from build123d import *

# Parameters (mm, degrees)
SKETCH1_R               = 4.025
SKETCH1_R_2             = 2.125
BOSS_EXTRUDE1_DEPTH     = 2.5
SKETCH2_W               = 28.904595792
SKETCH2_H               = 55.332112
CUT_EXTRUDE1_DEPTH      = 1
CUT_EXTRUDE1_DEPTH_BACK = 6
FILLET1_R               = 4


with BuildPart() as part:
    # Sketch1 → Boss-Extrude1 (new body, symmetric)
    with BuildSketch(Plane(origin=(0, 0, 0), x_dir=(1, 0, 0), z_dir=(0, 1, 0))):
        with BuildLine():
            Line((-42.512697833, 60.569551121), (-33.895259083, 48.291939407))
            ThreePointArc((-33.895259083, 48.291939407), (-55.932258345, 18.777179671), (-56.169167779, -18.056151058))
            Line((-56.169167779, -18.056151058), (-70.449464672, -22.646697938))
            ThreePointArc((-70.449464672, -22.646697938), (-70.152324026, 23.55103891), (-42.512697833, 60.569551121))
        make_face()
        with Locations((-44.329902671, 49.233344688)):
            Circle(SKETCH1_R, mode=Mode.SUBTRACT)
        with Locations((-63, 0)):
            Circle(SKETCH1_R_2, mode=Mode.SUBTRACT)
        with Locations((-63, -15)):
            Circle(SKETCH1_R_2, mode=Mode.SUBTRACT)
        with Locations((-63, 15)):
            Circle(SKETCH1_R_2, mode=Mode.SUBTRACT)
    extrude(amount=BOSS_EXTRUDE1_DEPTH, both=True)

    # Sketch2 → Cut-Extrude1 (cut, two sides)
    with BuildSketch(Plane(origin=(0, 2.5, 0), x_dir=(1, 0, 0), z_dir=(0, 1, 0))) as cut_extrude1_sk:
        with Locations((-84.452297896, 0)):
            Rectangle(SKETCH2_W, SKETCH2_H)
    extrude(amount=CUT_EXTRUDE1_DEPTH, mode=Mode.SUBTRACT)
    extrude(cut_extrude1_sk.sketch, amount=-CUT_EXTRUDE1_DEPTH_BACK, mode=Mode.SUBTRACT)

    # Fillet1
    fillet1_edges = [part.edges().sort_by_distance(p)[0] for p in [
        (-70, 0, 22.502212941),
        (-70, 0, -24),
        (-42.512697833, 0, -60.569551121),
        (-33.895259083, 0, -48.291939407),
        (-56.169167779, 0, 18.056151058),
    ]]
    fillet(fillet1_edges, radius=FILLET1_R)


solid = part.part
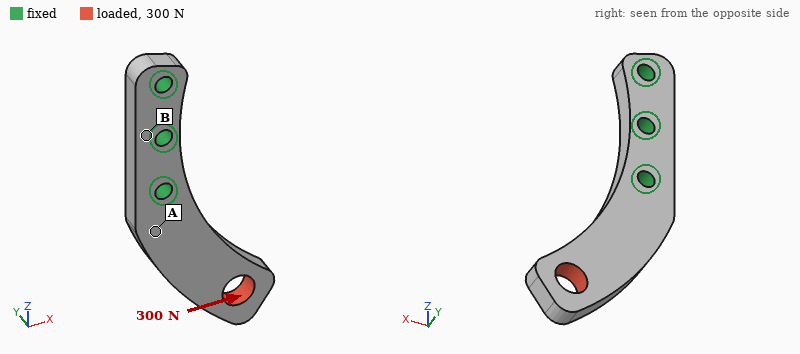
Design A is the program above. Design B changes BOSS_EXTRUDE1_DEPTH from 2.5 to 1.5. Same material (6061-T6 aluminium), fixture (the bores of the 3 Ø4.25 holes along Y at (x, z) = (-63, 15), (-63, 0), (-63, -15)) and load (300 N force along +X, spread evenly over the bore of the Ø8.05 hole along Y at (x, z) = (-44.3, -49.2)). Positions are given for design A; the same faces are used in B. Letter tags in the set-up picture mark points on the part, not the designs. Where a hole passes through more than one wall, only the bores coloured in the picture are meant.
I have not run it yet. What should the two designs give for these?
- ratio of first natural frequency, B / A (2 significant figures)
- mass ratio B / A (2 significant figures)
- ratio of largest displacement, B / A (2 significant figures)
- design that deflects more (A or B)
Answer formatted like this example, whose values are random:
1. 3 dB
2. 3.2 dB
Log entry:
1. 0.62
2. 0.60
3. 1.7
4. B
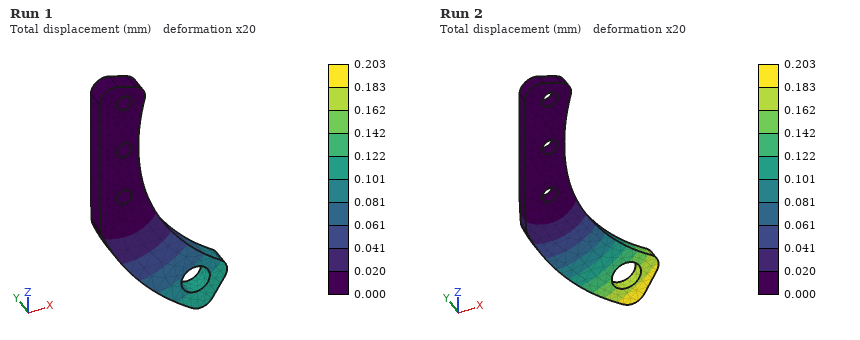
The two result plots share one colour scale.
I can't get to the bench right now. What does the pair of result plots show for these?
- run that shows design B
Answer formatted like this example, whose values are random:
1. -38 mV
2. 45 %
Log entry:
1. Run 2
